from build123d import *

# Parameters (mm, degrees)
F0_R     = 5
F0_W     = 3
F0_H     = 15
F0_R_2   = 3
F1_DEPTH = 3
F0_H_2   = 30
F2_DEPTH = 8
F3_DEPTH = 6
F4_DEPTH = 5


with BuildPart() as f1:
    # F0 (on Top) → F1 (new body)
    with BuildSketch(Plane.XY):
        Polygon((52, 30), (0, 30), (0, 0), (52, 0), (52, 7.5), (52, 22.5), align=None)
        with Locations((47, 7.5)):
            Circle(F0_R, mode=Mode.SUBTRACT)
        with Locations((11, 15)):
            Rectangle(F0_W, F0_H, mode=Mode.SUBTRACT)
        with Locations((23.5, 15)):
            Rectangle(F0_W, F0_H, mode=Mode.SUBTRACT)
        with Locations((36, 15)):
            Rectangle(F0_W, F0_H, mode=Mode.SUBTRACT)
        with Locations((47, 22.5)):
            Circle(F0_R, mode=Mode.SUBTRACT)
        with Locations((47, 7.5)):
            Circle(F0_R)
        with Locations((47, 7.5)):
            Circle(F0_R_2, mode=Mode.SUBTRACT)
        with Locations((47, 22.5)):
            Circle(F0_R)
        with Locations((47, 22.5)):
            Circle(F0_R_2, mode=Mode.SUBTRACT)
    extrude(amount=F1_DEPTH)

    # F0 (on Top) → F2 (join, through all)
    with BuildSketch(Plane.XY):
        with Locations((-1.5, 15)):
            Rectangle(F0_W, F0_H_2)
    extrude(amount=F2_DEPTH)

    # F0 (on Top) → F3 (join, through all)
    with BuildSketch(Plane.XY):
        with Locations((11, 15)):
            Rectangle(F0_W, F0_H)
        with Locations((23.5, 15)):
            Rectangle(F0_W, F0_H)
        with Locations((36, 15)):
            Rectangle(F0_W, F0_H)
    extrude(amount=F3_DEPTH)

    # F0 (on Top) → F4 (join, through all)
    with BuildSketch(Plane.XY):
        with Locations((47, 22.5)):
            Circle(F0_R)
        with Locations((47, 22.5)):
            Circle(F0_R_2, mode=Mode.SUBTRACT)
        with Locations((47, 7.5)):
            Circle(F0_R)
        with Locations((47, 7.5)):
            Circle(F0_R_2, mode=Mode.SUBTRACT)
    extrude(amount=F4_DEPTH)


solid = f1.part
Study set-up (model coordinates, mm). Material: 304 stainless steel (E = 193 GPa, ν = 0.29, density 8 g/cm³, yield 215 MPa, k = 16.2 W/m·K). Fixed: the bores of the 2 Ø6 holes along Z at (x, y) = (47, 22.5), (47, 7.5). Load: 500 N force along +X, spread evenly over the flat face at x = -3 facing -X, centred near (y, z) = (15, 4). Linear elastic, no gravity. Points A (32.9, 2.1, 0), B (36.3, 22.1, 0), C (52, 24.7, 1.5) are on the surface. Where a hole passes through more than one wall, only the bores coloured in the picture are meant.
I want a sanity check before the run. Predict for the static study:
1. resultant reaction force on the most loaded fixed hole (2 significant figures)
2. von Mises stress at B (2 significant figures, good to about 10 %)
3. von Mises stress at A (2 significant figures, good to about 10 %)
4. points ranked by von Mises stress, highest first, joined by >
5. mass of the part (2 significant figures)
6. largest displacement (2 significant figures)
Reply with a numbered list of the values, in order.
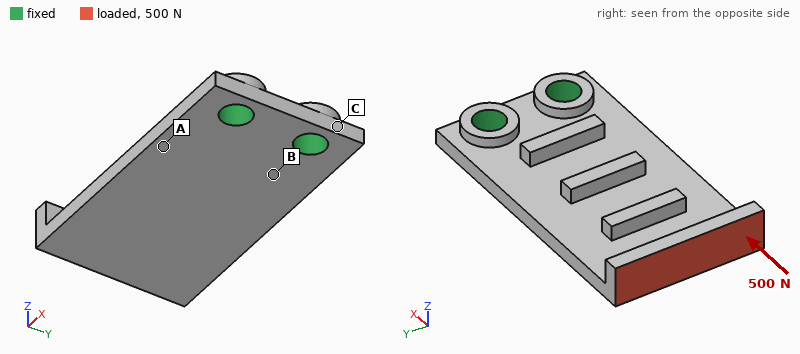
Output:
1. 250 N
2. 16 MPa
3. 21 MPa
4. A > B > C
5. 47 g
6. 0.10 mm
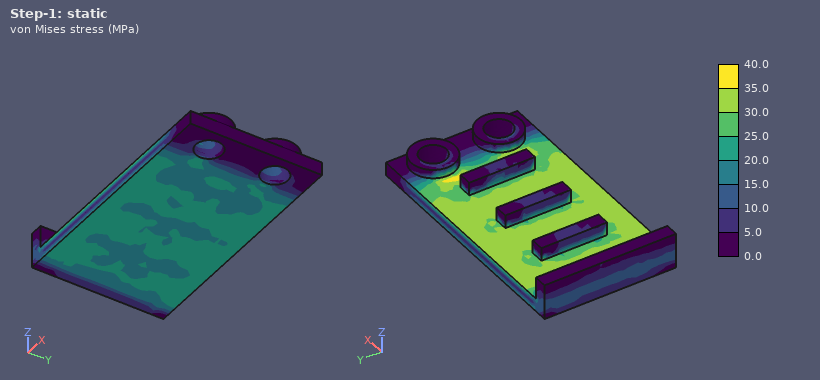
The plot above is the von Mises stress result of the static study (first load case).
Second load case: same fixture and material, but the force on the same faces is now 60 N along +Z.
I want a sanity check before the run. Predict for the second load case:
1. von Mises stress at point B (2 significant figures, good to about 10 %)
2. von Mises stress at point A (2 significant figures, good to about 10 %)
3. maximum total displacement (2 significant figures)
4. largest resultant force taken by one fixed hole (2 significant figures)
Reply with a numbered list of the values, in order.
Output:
1. 42 MPa
2. 46 MPa
3. 0.15 mm
4. 30 N
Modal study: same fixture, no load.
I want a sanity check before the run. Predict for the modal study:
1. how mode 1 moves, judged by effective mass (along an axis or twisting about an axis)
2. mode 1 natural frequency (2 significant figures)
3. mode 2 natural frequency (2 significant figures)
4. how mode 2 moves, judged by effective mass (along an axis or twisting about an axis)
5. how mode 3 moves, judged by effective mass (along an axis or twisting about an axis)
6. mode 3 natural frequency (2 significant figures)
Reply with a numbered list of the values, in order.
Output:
1. along Z
2. 920 Hz
3. 3400 Hz
4. twisting about X
5. along Z
6. 5700 Hz
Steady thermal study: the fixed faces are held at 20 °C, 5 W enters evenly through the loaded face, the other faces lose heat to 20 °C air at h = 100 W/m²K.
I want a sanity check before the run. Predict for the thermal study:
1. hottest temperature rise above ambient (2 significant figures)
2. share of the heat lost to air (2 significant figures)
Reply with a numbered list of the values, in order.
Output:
1. 43 K
2. 94 %
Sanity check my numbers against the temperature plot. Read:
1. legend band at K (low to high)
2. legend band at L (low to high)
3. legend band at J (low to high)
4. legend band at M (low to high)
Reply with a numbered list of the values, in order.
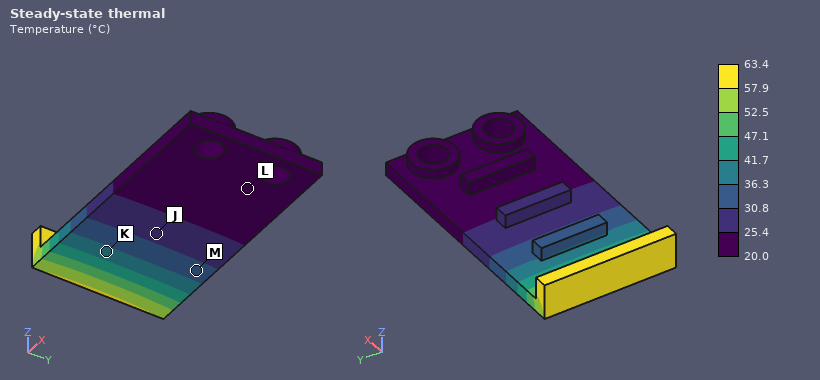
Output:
1. 36.3 to 41.7 °C
2. 20.0 to 25.4 °C
3. 25.4 to 30.8 °C
4. 30.8 to 36.3 °C
